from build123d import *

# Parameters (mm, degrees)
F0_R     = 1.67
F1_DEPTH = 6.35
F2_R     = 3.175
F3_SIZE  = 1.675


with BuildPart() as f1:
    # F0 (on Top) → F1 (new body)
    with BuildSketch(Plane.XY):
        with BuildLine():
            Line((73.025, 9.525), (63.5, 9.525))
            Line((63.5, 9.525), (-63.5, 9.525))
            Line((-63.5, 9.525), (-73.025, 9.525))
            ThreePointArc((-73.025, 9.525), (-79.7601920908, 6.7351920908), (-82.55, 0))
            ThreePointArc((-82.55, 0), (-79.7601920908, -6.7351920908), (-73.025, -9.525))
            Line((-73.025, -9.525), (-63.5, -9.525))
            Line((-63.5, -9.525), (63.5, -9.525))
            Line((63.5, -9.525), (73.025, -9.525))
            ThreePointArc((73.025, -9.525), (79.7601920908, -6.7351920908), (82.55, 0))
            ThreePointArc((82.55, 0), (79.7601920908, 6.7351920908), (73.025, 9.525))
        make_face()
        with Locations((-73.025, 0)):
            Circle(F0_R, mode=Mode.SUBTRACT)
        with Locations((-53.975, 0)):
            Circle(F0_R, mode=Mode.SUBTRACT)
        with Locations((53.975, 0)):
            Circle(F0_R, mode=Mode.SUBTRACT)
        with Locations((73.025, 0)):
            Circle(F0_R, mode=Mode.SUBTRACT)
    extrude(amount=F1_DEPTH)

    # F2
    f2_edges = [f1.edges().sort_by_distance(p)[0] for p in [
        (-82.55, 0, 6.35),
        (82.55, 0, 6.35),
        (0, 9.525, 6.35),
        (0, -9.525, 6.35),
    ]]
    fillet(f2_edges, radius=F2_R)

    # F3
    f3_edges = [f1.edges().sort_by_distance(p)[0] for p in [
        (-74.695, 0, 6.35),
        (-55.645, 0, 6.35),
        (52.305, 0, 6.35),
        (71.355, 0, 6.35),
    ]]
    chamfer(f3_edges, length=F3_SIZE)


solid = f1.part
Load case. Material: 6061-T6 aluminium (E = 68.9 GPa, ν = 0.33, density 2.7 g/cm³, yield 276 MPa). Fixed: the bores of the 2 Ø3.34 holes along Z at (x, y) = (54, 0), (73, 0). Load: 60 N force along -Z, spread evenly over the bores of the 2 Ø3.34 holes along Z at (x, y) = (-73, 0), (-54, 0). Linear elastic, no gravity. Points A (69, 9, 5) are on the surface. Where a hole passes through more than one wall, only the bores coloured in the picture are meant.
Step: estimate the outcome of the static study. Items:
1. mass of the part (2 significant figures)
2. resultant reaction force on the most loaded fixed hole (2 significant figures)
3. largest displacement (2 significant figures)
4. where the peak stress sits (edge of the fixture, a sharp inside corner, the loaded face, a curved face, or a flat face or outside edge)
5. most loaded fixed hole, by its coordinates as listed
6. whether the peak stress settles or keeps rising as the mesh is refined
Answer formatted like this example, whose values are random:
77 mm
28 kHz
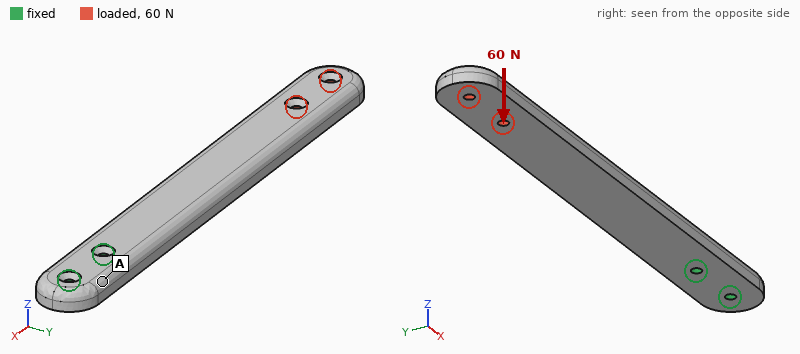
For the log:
50 g
250 N
1.6 mm
edge of the fixture
(54, 0)
keeps rising
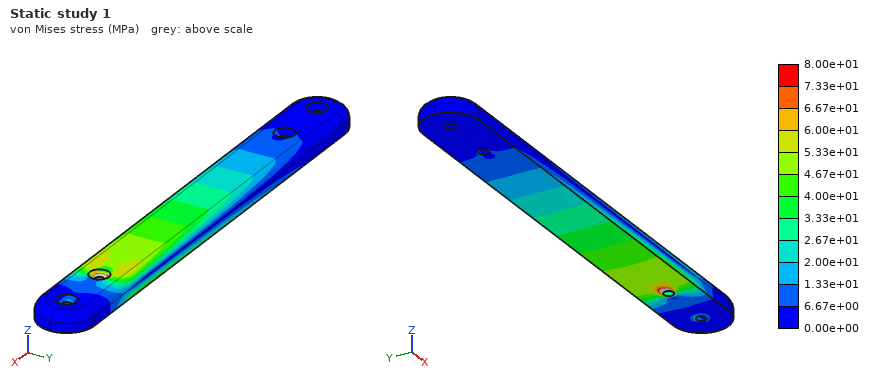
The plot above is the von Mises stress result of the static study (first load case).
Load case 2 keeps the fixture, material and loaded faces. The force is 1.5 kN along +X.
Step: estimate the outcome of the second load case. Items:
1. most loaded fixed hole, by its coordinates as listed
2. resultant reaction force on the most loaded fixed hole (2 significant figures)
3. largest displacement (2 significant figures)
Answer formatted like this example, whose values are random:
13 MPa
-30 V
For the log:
(54, 0)
1.2 kN
0.39 mm
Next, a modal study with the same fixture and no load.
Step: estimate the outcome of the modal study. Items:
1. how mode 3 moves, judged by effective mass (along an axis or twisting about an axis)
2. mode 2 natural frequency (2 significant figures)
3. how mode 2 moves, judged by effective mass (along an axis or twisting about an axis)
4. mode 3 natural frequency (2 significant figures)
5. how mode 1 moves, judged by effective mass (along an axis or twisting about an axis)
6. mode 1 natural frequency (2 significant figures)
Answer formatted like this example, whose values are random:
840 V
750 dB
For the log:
along Z
740 Hz
along Y
1700 Hz
along Z
280 Hz
